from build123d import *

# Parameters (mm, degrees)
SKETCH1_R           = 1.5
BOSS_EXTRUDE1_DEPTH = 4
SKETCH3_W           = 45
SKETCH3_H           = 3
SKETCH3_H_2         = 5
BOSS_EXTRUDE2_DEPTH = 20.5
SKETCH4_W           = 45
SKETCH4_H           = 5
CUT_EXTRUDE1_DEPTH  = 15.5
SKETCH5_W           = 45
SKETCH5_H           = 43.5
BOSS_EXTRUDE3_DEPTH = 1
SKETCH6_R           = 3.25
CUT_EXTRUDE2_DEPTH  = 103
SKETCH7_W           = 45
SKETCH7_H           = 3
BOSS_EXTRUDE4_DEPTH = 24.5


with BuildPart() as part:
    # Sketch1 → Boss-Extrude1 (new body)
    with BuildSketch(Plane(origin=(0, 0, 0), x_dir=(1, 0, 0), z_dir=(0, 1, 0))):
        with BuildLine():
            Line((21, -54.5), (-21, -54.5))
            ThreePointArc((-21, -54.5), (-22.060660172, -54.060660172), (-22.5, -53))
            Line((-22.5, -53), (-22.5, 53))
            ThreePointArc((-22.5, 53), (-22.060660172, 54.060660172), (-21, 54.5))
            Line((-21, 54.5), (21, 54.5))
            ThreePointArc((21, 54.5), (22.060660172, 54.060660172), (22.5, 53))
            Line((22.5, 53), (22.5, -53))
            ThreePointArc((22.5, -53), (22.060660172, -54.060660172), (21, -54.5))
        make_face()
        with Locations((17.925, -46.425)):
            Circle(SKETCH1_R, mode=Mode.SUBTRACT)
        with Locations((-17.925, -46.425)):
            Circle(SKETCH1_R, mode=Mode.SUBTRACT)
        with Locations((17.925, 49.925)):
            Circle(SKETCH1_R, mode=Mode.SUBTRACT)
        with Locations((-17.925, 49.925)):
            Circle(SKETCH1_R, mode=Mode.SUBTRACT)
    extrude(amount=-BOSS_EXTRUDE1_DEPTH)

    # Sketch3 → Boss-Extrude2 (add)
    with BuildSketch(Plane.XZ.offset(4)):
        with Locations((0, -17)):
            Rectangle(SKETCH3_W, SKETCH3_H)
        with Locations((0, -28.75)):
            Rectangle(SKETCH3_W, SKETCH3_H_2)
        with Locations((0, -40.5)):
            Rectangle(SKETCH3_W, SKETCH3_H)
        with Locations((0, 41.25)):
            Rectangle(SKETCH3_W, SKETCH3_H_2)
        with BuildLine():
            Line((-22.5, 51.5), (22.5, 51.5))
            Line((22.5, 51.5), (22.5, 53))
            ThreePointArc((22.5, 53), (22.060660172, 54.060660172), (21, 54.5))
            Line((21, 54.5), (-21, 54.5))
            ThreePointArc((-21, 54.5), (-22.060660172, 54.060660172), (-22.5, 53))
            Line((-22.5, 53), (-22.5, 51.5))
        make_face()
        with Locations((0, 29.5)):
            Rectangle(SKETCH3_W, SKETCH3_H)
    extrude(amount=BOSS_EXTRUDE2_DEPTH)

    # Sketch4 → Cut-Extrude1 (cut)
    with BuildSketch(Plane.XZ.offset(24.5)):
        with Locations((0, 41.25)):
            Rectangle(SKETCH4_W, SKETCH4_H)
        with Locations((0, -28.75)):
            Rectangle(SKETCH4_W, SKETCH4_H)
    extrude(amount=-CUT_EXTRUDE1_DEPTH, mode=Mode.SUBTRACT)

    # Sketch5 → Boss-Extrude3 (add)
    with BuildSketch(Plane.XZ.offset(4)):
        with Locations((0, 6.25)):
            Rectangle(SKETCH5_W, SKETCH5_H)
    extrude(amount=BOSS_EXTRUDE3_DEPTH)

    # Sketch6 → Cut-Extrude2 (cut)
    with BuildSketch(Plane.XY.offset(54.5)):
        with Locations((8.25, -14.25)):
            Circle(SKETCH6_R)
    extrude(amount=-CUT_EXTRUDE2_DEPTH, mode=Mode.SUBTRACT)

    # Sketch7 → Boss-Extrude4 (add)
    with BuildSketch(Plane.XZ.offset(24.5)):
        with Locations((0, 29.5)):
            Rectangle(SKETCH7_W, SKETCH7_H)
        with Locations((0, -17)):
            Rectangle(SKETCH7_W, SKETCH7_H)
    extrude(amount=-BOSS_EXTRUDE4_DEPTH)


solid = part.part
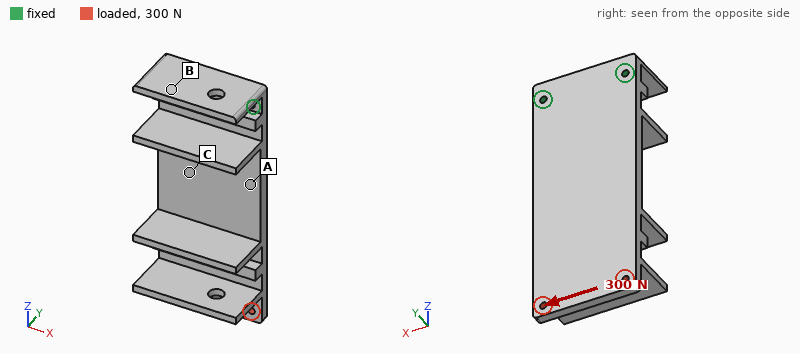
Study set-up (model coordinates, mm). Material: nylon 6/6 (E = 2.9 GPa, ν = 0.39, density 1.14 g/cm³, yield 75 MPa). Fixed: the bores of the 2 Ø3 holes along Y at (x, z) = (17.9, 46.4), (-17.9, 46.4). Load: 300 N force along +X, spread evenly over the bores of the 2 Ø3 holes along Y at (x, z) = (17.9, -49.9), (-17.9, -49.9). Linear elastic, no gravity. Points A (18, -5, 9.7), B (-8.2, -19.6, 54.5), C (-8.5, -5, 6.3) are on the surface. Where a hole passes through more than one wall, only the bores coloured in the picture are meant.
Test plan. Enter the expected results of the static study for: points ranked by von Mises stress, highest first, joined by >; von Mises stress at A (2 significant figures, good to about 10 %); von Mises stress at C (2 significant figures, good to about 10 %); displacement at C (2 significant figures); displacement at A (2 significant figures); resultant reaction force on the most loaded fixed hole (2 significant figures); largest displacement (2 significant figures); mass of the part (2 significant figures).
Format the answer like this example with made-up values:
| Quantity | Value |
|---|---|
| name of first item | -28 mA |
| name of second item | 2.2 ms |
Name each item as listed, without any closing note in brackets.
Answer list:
| Quantity | Value |
|---|---|
| points ranked by von Mises stress, highest first, joined by > | A > C > B |
| von Mises stress at A | 8.0 MPa |
| von Mises stress at C | 4.1 MPa |
| displacement at C | 0.29 mm |
| displacement at A | 0.32 mm |
| resultant reaction force on the most loaded fixed hole | 810 N |
| largest displacement | 1.2 mm |
| mass of the part | 39 g |
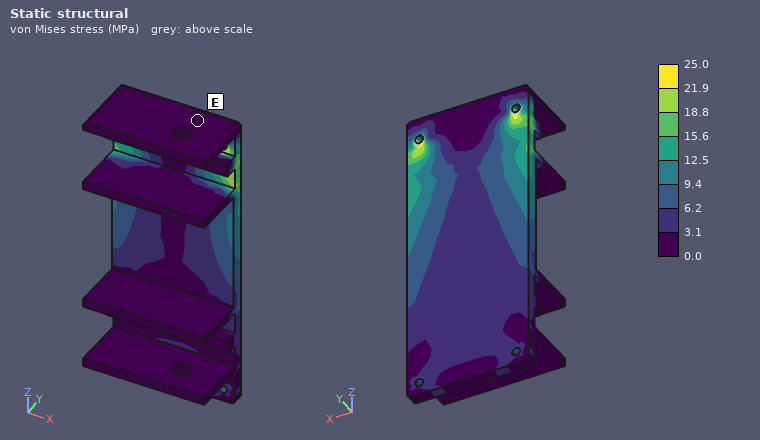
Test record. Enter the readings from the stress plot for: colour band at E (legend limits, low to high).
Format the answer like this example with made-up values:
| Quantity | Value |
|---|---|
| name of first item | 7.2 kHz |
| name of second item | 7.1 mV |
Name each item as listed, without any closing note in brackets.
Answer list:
| Quantity | Value |
|---|---|
| colour band at E | 0.0 to 3.1 MPa |
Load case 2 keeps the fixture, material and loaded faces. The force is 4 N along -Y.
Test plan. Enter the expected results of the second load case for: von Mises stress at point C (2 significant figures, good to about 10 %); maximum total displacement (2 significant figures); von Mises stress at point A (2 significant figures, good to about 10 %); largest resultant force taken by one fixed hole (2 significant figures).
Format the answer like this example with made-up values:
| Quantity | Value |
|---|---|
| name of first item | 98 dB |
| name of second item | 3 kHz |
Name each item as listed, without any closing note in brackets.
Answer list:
| Quantity | Value |
|---|---|
| von Mises stress at point C | 1.1 MPa |
| maximum total displacement | 1.2 mm |
| von Mises stress at point A | 1.2 MPa |
| largest resultant force taken by one fixed hole | 2.7 N |
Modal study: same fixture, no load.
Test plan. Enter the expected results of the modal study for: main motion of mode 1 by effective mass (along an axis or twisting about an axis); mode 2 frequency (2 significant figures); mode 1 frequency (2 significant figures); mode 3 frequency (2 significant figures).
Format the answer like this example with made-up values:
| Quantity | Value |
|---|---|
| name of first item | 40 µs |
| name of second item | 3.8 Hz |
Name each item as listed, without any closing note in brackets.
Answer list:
| Quantity | Value |
|---|---|
| main motion of mode 1 by effective mass | along Y |
| mode 2 frequency | 420 Hz |
| mode 1 frequency | 92 Hz |
| mode 3 frequency | 580 Hz |
